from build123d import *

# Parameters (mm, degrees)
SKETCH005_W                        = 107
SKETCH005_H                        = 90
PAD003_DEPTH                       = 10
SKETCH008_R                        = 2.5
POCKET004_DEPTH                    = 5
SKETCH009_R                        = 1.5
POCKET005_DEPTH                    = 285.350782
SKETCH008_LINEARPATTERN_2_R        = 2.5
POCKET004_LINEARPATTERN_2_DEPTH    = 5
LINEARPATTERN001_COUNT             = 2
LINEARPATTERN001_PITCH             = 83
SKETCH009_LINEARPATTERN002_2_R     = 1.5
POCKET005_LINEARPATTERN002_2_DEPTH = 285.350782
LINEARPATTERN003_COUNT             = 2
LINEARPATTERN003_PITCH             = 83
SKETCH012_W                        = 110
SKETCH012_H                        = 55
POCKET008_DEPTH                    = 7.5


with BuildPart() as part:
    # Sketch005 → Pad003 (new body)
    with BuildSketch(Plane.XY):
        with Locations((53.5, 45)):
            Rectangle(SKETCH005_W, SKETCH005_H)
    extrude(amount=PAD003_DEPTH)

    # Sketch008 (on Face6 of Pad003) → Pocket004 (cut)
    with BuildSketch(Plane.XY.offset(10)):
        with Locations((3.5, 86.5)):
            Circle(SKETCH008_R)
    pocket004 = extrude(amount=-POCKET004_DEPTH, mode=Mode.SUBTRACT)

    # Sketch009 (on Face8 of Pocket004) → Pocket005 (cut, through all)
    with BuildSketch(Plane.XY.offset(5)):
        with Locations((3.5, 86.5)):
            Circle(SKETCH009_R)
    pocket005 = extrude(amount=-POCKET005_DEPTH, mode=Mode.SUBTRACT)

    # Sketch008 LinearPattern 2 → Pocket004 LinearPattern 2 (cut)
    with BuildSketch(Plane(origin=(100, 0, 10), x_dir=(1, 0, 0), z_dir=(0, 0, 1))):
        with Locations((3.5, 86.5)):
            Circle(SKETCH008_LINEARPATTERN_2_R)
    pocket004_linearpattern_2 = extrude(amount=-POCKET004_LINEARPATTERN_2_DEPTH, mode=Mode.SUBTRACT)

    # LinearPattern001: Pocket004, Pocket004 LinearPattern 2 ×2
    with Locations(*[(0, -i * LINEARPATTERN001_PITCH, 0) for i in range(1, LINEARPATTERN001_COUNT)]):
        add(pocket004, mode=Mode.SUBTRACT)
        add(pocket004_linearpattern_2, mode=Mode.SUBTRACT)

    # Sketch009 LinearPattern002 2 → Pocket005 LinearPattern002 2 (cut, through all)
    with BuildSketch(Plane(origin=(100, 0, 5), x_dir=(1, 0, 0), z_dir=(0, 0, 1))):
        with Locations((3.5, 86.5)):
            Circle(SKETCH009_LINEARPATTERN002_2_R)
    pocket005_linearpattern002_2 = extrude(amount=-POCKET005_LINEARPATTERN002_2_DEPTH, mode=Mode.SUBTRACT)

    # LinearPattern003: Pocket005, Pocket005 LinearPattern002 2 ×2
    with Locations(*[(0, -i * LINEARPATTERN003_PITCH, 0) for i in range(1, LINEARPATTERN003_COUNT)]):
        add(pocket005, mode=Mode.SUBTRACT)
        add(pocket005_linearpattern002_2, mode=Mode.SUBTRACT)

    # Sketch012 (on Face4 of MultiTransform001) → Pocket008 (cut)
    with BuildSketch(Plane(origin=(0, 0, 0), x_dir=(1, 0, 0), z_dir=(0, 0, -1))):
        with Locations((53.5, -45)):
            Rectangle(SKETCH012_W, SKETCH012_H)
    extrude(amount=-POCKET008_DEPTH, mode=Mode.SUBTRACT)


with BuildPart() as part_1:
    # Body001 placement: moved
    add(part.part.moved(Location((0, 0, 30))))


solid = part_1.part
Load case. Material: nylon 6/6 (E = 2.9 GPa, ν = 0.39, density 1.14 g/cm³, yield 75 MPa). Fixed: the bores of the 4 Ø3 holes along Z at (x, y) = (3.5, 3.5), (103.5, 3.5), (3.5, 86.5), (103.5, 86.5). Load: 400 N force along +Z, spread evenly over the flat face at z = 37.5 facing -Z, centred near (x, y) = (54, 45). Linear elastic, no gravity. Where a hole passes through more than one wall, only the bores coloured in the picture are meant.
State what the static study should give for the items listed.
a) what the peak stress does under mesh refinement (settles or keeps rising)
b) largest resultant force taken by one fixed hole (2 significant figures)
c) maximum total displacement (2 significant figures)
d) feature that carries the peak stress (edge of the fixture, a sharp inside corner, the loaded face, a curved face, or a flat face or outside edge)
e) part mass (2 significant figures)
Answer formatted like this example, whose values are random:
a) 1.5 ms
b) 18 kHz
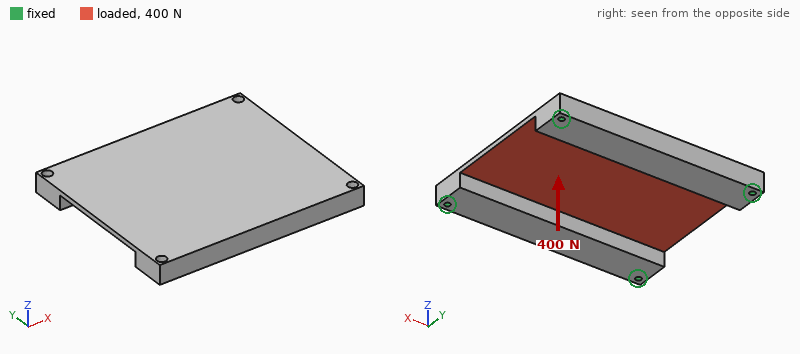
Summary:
a) keeps rising
b) 320 N
c) 0.84 mm
d) edge of the fixture
e) 59 g
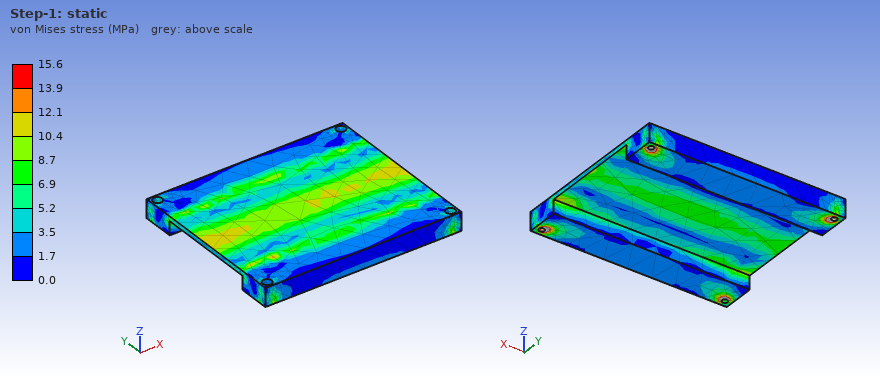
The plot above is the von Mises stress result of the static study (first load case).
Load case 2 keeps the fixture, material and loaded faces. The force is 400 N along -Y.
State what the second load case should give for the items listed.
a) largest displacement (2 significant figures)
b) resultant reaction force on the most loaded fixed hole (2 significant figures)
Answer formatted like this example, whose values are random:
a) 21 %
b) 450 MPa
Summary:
a) 99 µm
b) 110 N
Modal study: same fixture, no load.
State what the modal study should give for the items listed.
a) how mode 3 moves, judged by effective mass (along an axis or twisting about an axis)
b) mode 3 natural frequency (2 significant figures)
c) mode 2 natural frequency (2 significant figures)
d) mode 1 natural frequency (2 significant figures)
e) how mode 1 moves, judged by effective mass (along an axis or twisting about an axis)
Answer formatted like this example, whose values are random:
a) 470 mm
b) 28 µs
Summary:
a) twisting about Y
b) 1300 Hz
c) 1000 Hz
d) 890 Hz
e) along Z
